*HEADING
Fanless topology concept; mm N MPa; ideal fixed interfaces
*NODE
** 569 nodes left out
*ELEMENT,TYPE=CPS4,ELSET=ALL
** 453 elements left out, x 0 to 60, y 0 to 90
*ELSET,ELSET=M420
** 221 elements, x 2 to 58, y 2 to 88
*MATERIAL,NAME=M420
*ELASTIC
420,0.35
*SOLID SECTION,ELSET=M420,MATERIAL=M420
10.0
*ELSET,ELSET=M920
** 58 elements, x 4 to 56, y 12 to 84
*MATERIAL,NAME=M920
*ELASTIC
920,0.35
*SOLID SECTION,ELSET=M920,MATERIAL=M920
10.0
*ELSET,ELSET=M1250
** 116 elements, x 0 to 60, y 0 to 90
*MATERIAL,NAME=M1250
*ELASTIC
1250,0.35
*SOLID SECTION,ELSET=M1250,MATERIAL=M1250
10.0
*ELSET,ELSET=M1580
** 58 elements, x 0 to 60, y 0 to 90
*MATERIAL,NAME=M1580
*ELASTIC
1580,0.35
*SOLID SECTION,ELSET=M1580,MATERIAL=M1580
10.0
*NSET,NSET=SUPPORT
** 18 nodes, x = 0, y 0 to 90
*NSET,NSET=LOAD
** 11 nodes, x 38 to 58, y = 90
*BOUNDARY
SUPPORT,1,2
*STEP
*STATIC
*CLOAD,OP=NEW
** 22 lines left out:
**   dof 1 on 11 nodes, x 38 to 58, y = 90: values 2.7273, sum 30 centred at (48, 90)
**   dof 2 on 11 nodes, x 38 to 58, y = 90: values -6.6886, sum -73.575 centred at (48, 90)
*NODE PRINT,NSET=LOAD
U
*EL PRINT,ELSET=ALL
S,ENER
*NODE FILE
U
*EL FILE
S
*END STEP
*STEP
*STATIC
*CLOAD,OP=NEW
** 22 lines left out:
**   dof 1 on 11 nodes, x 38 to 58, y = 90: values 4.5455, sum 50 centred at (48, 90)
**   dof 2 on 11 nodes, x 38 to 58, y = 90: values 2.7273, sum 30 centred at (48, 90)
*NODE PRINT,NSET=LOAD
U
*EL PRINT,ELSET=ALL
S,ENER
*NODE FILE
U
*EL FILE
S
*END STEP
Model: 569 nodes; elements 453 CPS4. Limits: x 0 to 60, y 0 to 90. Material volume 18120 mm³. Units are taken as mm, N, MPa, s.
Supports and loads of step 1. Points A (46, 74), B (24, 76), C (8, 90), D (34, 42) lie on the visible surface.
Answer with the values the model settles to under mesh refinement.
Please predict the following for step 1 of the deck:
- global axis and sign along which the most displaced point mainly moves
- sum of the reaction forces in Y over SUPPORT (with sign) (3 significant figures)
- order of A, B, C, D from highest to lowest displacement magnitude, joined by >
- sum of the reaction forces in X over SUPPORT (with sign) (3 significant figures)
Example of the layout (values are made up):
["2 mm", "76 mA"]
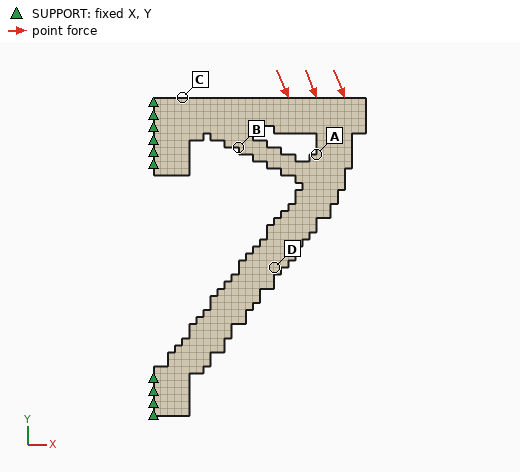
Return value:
["-Y", "73.6 N", "A > D > B > C", "-30.0 N"]
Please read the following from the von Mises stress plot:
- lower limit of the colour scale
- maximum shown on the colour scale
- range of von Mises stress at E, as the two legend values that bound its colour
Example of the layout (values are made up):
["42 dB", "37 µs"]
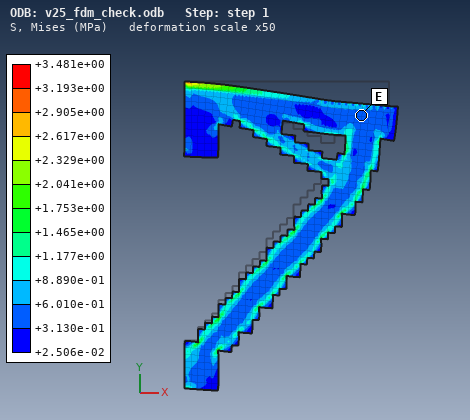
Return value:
["+2.506e-02 MPa", "+3.481e+00 MPa", "+3.130e-01 to +6.010e-01 MPa"]
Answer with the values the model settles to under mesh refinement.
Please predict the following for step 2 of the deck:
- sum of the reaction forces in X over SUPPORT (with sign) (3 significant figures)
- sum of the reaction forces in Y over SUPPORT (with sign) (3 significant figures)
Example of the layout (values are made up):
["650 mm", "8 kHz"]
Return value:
["-50.0 N", "-30.0 N"]
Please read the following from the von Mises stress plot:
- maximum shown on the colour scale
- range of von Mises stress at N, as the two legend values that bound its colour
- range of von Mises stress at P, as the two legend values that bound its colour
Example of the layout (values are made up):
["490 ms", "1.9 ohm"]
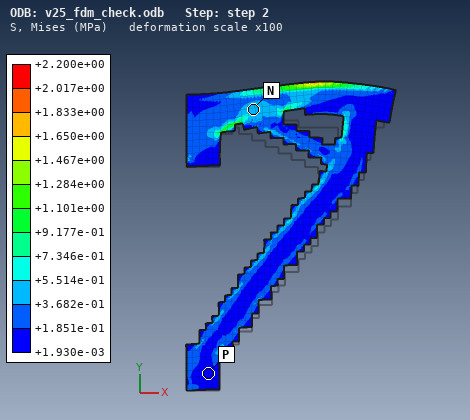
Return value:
["+2.200e+00 MPa", "+3.682e-01 to +5.514e-01 MPa", "+1.930e-03 to +1.851e-01 MPa"]
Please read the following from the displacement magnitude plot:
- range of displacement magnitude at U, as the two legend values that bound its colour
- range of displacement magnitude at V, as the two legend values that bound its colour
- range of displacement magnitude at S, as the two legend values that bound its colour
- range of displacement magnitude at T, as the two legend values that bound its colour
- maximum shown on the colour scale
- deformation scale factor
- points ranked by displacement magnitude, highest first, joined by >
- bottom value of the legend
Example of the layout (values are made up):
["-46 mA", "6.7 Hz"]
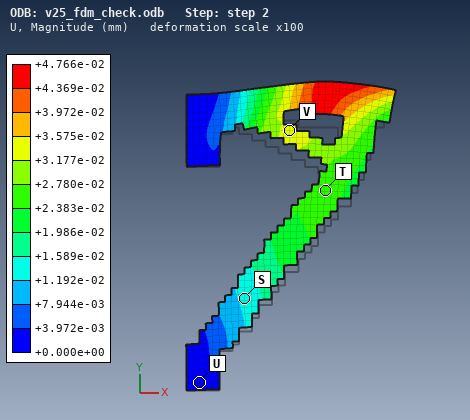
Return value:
["+0.000e+00 to +3.972e-03 mm", "+3.177e-02 to +3.575e-02 mm", "+1.192e-02 to +1.589e-02 mm", "+2.383e-02 to +2.780e-02 mm", "+4.766e-02 mm", "100", "V > T > S > U", "+0.000e+00 mm"]
